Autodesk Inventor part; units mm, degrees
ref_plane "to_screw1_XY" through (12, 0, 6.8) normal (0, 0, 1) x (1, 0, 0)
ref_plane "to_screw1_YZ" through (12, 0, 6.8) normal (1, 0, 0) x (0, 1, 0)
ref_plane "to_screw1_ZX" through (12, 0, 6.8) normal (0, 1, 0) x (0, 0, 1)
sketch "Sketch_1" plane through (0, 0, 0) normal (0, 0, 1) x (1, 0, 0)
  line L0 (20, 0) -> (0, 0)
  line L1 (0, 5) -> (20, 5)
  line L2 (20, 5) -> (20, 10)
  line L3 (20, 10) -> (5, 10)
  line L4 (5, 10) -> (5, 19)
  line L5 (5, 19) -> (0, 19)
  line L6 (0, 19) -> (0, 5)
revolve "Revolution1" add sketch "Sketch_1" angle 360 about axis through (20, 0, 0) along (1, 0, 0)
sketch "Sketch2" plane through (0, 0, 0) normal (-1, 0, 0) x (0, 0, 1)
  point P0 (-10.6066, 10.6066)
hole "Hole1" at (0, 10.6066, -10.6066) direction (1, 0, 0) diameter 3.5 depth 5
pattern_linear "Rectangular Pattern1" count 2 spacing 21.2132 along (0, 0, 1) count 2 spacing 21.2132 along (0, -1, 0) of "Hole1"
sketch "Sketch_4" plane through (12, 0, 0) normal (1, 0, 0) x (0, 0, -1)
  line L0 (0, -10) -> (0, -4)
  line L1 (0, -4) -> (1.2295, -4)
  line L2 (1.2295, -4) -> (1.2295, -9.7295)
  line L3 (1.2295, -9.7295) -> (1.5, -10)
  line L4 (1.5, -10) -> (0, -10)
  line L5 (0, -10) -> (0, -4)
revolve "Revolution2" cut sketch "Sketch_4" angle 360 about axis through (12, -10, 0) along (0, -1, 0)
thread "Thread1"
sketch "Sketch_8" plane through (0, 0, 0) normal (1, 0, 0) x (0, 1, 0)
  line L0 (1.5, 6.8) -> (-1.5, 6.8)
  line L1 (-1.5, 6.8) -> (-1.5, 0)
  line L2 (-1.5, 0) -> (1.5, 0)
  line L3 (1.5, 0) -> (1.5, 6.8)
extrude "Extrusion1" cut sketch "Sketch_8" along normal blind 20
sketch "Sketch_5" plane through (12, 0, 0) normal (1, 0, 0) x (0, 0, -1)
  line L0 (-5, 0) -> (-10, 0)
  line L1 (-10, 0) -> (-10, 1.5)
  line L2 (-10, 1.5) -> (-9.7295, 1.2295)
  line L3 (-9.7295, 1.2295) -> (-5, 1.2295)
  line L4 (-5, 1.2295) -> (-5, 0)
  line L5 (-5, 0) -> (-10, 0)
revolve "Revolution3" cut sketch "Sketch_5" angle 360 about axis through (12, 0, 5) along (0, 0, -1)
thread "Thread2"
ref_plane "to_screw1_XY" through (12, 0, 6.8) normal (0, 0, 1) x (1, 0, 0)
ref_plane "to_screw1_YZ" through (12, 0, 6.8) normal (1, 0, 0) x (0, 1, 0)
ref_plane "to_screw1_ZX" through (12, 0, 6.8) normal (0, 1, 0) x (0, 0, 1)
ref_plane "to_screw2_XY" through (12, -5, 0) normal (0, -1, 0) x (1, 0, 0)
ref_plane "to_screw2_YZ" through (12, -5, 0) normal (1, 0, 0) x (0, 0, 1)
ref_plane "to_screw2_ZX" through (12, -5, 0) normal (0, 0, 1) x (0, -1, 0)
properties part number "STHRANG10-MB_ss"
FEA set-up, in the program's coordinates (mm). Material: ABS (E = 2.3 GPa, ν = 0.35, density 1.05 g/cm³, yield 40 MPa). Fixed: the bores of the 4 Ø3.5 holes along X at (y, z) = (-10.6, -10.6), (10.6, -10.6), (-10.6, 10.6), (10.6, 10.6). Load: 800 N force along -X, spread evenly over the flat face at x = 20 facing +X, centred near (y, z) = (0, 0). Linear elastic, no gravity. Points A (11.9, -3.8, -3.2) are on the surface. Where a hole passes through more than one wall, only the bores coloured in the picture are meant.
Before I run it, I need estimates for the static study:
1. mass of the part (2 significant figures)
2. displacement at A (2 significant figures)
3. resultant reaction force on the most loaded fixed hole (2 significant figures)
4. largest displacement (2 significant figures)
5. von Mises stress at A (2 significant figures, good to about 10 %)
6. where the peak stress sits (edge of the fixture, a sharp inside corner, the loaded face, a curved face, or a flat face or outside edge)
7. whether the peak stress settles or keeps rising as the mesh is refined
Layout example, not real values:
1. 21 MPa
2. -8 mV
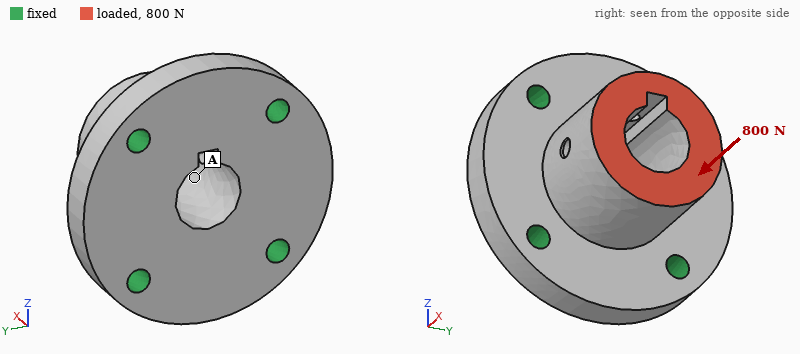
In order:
1. 8.9 g
2. 55 µm
3. 210 N
4. 72 µm
5. 3.4 MPa
6. edge of the fixture
7. keeps rising
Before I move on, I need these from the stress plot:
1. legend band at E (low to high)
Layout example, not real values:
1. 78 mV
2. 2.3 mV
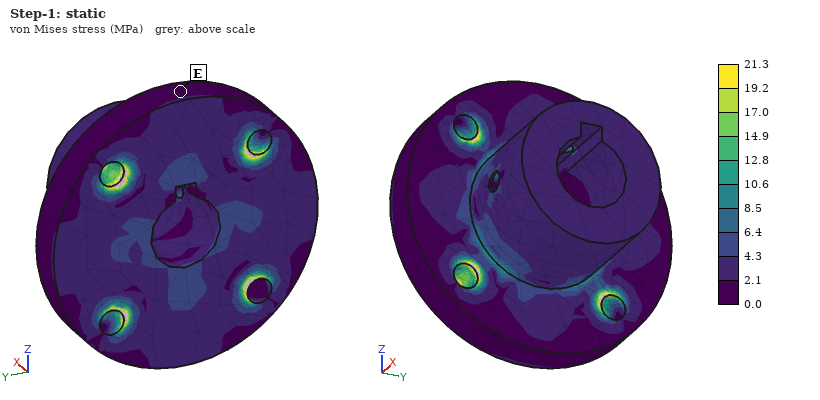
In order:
1. 0.0 to 2.1 MPa
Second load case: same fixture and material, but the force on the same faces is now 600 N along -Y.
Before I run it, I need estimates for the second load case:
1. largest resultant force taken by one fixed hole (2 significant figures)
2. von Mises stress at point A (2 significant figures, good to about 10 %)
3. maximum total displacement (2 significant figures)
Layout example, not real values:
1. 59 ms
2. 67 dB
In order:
1. 320 N
2. 8.5 MPa
3. 0.31 mm
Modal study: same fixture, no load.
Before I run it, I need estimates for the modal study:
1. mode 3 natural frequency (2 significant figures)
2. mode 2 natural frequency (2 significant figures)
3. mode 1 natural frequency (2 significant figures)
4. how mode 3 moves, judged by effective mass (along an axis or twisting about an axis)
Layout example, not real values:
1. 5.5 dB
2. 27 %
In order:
1. 8500 Hz
2. 6300 Hz
3. 6200 Hz
4. along X
